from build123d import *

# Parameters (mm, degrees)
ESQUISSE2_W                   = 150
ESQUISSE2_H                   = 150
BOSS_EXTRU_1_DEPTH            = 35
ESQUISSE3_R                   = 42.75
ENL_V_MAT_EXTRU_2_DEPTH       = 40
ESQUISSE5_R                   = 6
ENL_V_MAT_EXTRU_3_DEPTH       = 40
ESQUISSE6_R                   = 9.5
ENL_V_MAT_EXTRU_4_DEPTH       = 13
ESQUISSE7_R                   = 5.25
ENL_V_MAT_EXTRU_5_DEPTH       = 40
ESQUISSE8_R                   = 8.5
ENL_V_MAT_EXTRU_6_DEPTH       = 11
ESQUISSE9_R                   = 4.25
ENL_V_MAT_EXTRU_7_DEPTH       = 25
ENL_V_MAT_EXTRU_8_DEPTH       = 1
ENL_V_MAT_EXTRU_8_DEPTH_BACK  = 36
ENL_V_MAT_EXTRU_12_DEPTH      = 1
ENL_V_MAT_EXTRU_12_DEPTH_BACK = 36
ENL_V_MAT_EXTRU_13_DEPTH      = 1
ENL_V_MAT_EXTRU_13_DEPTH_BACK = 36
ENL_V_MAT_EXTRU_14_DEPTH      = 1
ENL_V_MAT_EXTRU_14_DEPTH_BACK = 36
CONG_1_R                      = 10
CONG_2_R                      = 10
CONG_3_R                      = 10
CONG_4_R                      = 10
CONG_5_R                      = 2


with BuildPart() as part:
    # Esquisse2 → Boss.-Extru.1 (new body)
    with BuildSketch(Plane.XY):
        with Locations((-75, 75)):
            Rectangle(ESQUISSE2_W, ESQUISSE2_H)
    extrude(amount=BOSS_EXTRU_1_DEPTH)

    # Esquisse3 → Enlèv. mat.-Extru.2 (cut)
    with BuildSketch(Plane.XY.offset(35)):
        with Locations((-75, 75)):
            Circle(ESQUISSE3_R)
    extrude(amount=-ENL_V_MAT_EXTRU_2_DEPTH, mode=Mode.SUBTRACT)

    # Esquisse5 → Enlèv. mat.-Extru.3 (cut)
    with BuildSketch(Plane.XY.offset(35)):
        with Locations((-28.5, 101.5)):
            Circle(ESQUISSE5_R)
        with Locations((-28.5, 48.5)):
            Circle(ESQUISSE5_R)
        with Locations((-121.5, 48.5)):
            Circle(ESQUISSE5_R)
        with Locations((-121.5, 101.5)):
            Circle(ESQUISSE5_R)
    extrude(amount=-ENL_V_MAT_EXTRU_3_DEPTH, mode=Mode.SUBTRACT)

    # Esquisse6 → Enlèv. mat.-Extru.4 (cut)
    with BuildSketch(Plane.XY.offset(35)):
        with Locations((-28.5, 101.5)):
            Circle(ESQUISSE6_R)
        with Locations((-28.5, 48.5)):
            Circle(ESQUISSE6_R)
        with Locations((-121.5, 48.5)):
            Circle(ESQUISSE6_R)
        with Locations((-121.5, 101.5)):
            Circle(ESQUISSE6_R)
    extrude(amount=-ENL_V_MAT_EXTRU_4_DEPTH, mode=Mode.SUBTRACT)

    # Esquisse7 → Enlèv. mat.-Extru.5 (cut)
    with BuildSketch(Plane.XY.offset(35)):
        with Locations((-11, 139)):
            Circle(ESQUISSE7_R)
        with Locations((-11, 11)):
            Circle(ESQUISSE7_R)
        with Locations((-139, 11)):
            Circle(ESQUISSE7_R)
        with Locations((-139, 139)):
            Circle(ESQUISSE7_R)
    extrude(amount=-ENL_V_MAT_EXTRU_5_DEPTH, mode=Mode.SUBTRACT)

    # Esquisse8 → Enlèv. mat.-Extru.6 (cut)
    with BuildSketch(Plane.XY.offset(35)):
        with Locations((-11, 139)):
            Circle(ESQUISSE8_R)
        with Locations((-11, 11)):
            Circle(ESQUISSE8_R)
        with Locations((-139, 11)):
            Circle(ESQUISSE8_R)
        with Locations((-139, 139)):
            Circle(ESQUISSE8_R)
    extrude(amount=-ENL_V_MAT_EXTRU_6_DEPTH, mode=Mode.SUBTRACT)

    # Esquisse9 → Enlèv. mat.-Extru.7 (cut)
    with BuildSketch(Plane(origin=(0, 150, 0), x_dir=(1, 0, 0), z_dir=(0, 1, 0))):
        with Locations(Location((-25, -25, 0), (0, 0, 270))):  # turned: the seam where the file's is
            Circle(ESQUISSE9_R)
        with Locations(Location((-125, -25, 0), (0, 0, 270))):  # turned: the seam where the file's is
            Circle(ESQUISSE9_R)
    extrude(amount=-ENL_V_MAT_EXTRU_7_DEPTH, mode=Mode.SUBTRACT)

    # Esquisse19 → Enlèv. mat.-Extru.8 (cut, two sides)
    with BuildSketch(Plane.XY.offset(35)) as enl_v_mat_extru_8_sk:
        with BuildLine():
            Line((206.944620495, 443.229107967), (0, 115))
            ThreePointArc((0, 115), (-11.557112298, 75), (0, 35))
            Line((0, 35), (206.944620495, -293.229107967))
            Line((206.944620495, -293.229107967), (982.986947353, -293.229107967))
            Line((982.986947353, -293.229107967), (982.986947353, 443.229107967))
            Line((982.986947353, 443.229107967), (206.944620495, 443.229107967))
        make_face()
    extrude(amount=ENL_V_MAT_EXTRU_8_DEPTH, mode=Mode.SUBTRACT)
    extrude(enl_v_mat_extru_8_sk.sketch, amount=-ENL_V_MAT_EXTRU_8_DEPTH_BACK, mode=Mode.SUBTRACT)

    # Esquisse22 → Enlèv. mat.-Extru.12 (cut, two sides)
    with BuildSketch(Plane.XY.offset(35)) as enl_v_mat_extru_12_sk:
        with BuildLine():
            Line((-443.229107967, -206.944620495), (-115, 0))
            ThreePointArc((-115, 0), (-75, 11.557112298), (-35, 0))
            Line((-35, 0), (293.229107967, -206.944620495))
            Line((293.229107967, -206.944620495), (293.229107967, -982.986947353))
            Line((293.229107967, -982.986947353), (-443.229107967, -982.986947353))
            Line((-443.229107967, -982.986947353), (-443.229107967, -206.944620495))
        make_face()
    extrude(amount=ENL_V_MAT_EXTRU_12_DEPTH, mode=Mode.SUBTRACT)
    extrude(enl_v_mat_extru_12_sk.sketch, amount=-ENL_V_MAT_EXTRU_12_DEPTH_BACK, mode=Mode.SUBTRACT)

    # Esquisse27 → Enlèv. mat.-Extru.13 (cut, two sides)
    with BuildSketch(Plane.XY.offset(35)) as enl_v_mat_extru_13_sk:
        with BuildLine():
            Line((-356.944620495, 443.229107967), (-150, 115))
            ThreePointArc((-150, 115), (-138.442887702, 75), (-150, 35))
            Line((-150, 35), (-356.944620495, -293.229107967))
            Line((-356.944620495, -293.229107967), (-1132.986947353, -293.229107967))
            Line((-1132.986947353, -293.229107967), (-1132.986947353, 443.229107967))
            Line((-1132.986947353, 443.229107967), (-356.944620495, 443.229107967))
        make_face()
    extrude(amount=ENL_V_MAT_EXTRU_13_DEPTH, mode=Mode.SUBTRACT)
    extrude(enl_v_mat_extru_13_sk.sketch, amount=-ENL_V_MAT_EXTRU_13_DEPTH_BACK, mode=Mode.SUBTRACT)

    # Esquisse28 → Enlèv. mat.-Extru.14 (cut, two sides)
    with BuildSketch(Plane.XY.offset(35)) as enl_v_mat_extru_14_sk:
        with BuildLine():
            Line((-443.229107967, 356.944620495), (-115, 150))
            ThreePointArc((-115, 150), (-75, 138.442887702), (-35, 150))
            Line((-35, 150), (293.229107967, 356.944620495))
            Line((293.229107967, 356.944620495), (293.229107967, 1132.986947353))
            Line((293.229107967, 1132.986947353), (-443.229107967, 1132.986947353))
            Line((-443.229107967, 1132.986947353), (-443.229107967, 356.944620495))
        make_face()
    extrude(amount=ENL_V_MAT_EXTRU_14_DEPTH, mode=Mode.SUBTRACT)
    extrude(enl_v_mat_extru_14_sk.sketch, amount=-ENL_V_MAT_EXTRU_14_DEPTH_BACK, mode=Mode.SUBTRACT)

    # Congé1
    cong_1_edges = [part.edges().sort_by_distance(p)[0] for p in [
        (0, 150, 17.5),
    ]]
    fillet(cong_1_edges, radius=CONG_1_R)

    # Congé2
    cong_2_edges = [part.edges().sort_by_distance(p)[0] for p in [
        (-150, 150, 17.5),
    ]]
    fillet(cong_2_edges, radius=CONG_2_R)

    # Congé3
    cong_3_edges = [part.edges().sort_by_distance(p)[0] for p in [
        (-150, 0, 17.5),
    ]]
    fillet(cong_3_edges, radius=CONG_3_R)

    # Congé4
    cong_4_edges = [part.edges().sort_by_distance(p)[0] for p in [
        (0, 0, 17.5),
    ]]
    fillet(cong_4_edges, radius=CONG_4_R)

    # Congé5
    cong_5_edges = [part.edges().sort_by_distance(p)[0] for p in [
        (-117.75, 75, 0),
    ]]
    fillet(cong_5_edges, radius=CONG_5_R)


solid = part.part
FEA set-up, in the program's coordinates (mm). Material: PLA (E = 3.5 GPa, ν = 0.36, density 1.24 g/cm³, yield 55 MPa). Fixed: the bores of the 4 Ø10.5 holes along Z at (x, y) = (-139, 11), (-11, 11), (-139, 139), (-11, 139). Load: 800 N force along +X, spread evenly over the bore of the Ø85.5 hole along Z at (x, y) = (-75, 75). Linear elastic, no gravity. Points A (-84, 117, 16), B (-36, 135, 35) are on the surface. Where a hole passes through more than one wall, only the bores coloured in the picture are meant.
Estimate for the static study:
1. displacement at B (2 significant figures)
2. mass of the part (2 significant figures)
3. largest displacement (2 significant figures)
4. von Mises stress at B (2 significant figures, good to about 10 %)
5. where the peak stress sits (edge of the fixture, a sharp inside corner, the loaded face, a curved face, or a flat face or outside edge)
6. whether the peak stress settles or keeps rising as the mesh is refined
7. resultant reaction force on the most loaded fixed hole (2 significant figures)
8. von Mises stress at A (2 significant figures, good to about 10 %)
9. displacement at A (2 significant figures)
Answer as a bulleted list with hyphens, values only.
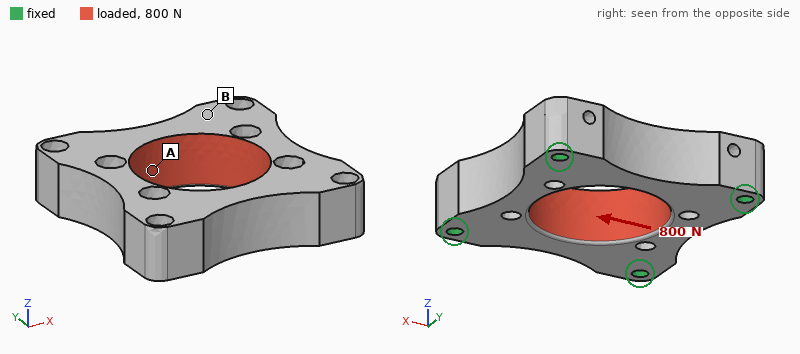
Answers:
- 2.9 µm
- 560 g
- 12 µm
- 0.092 MPa
- edge of the fixture
- keeps rising
- 230 N
- 0.29 MPa
- 3.7 µm
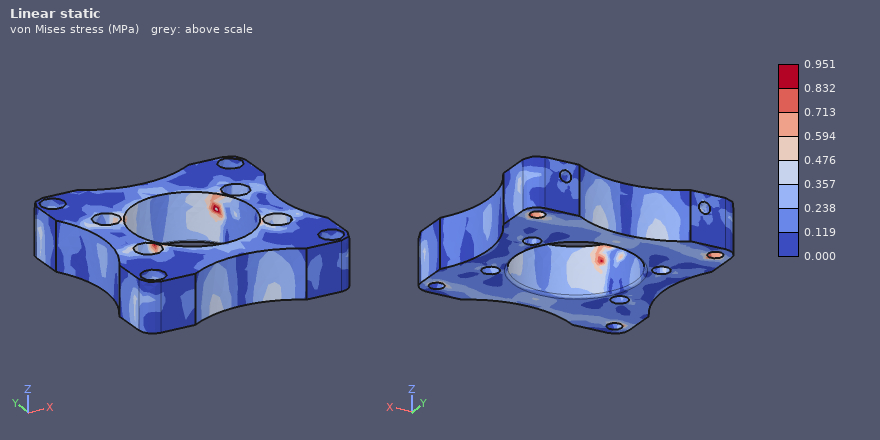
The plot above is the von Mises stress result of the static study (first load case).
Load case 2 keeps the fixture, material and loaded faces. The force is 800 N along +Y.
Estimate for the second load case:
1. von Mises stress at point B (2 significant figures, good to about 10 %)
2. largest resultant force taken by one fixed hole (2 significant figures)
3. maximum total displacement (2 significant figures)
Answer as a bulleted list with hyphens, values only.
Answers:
- 0.12 MPa
- 230 N
- 11 µm
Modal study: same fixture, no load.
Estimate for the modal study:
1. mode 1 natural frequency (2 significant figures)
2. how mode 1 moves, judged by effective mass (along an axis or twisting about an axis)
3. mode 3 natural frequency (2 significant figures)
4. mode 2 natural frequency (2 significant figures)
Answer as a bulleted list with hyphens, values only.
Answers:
- 1800 Hz
- along Z
- 2400 Hz
- 1900 Hz
